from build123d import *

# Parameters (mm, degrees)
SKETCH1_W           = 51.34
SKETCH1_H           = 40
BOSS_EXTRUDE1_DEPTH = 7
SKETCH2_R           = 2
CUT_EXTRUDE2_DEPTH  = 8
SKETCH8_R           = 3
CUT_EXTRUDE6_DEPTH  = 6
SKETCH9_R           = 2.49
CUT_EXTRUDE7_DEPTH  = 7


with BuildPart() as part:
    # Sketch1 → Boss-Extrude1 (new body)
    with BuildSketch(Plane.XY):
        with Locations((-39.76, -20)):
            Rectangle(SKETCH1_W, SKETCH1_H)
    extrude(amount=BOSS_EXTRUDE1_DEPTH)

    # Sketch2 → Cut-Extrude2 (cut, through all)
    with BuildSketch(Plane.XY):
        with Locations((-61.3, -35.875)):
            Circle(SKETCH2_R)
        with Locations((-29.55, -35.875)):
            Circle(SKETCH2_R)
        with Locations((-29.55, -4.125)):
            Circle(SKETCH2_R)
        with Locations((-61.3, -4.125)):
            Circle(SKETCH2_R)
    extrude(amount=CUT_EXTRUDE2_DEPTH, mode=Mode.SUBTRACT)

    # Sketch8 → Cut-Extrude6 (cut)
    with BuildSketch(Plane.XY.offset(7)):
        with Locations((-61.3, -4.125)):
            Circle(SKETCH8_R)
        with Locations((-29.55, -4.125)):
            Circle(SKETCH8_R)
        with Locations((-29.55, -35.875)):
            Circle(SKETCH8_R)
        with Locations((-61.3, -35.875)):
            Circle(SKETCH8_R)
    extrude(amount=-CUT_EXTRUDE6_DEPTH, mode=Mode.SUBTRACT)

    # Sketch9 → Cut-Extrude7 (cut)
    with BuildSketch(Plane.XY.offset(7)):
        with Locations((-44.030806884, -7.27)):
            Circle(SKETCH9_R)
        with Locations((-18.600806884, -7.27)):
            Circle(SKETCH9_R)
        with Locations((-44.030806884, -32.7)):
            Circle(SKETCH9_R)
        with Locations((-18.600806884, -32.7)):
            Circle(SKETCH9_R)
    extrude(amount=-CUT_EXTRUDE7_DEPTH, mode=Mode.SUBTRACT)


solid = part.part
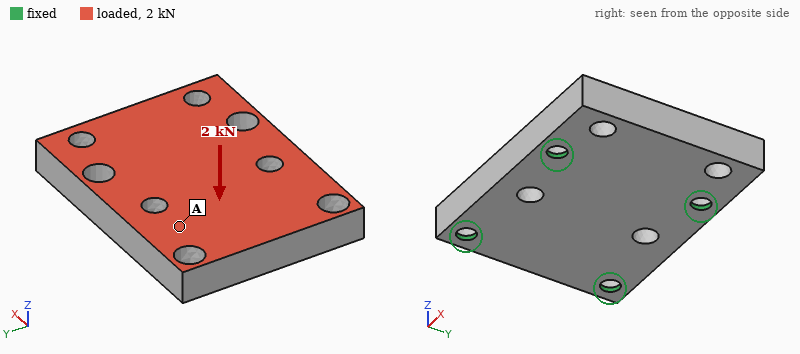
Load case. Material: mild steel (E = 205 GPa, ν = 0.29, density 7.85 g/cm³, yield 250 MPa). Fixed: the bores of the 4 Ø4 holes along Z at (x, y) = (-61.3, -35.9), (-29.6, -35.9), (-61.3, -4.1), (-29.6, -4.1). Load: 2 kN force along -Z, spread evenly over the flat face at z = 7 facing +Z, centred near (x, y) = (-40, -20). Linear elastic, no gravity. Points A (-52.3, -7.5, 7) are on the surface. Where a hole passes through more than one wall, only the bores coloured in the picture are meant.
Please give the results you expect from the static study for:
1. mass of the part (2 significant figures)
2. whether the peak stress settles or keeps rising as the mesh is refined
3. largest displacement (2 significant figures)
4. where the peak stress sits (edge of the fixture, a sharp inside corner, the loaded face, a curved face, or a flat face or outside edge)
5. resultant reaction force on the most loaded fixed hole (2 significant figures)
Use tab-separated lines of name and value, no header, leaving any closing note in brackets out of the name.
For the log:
mass of the part	100 g
whether the peak stress settles or keeps rising as the mesh is refined	keeps rising
largest displacement	5.9 µm
where the peak stress sits	edge of the fixture
resultant reaction force on the most loaded fixed hole	750 N
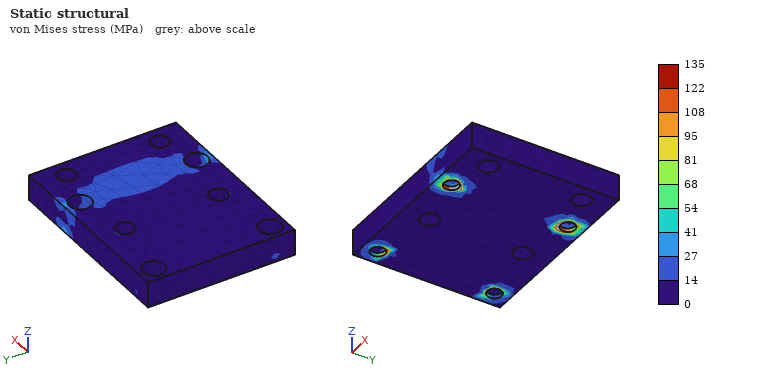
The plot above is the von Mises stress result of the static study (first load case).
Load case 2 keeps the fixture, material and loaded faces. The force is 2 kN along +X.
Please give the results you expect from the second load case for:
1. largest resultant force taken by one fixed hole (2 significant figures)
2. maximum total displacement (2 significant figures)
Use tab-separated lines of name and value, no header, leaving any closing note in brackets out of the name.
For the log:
largest resultant force taken by one fixed hole	560 N
maximum total displacement	5.3 µm
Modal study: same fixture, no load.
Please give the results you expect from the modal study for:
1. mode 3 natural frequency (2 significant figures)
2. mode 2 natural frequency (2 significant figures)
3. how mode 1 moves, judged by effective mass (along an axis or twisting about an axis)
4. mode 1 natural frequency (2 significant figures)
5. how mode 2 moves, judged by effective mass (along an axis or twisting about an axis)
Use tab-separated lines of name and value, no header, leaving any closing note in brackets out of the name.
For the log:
mode 3 natural frequency	19 kHz
mode 2 natural frequency	14 kHz
how mode 1 moves, judged by effective mass	along Z
mode 1 natural frequency	11 kHz
how mode 2 moves, judged by effective mass	along Z
